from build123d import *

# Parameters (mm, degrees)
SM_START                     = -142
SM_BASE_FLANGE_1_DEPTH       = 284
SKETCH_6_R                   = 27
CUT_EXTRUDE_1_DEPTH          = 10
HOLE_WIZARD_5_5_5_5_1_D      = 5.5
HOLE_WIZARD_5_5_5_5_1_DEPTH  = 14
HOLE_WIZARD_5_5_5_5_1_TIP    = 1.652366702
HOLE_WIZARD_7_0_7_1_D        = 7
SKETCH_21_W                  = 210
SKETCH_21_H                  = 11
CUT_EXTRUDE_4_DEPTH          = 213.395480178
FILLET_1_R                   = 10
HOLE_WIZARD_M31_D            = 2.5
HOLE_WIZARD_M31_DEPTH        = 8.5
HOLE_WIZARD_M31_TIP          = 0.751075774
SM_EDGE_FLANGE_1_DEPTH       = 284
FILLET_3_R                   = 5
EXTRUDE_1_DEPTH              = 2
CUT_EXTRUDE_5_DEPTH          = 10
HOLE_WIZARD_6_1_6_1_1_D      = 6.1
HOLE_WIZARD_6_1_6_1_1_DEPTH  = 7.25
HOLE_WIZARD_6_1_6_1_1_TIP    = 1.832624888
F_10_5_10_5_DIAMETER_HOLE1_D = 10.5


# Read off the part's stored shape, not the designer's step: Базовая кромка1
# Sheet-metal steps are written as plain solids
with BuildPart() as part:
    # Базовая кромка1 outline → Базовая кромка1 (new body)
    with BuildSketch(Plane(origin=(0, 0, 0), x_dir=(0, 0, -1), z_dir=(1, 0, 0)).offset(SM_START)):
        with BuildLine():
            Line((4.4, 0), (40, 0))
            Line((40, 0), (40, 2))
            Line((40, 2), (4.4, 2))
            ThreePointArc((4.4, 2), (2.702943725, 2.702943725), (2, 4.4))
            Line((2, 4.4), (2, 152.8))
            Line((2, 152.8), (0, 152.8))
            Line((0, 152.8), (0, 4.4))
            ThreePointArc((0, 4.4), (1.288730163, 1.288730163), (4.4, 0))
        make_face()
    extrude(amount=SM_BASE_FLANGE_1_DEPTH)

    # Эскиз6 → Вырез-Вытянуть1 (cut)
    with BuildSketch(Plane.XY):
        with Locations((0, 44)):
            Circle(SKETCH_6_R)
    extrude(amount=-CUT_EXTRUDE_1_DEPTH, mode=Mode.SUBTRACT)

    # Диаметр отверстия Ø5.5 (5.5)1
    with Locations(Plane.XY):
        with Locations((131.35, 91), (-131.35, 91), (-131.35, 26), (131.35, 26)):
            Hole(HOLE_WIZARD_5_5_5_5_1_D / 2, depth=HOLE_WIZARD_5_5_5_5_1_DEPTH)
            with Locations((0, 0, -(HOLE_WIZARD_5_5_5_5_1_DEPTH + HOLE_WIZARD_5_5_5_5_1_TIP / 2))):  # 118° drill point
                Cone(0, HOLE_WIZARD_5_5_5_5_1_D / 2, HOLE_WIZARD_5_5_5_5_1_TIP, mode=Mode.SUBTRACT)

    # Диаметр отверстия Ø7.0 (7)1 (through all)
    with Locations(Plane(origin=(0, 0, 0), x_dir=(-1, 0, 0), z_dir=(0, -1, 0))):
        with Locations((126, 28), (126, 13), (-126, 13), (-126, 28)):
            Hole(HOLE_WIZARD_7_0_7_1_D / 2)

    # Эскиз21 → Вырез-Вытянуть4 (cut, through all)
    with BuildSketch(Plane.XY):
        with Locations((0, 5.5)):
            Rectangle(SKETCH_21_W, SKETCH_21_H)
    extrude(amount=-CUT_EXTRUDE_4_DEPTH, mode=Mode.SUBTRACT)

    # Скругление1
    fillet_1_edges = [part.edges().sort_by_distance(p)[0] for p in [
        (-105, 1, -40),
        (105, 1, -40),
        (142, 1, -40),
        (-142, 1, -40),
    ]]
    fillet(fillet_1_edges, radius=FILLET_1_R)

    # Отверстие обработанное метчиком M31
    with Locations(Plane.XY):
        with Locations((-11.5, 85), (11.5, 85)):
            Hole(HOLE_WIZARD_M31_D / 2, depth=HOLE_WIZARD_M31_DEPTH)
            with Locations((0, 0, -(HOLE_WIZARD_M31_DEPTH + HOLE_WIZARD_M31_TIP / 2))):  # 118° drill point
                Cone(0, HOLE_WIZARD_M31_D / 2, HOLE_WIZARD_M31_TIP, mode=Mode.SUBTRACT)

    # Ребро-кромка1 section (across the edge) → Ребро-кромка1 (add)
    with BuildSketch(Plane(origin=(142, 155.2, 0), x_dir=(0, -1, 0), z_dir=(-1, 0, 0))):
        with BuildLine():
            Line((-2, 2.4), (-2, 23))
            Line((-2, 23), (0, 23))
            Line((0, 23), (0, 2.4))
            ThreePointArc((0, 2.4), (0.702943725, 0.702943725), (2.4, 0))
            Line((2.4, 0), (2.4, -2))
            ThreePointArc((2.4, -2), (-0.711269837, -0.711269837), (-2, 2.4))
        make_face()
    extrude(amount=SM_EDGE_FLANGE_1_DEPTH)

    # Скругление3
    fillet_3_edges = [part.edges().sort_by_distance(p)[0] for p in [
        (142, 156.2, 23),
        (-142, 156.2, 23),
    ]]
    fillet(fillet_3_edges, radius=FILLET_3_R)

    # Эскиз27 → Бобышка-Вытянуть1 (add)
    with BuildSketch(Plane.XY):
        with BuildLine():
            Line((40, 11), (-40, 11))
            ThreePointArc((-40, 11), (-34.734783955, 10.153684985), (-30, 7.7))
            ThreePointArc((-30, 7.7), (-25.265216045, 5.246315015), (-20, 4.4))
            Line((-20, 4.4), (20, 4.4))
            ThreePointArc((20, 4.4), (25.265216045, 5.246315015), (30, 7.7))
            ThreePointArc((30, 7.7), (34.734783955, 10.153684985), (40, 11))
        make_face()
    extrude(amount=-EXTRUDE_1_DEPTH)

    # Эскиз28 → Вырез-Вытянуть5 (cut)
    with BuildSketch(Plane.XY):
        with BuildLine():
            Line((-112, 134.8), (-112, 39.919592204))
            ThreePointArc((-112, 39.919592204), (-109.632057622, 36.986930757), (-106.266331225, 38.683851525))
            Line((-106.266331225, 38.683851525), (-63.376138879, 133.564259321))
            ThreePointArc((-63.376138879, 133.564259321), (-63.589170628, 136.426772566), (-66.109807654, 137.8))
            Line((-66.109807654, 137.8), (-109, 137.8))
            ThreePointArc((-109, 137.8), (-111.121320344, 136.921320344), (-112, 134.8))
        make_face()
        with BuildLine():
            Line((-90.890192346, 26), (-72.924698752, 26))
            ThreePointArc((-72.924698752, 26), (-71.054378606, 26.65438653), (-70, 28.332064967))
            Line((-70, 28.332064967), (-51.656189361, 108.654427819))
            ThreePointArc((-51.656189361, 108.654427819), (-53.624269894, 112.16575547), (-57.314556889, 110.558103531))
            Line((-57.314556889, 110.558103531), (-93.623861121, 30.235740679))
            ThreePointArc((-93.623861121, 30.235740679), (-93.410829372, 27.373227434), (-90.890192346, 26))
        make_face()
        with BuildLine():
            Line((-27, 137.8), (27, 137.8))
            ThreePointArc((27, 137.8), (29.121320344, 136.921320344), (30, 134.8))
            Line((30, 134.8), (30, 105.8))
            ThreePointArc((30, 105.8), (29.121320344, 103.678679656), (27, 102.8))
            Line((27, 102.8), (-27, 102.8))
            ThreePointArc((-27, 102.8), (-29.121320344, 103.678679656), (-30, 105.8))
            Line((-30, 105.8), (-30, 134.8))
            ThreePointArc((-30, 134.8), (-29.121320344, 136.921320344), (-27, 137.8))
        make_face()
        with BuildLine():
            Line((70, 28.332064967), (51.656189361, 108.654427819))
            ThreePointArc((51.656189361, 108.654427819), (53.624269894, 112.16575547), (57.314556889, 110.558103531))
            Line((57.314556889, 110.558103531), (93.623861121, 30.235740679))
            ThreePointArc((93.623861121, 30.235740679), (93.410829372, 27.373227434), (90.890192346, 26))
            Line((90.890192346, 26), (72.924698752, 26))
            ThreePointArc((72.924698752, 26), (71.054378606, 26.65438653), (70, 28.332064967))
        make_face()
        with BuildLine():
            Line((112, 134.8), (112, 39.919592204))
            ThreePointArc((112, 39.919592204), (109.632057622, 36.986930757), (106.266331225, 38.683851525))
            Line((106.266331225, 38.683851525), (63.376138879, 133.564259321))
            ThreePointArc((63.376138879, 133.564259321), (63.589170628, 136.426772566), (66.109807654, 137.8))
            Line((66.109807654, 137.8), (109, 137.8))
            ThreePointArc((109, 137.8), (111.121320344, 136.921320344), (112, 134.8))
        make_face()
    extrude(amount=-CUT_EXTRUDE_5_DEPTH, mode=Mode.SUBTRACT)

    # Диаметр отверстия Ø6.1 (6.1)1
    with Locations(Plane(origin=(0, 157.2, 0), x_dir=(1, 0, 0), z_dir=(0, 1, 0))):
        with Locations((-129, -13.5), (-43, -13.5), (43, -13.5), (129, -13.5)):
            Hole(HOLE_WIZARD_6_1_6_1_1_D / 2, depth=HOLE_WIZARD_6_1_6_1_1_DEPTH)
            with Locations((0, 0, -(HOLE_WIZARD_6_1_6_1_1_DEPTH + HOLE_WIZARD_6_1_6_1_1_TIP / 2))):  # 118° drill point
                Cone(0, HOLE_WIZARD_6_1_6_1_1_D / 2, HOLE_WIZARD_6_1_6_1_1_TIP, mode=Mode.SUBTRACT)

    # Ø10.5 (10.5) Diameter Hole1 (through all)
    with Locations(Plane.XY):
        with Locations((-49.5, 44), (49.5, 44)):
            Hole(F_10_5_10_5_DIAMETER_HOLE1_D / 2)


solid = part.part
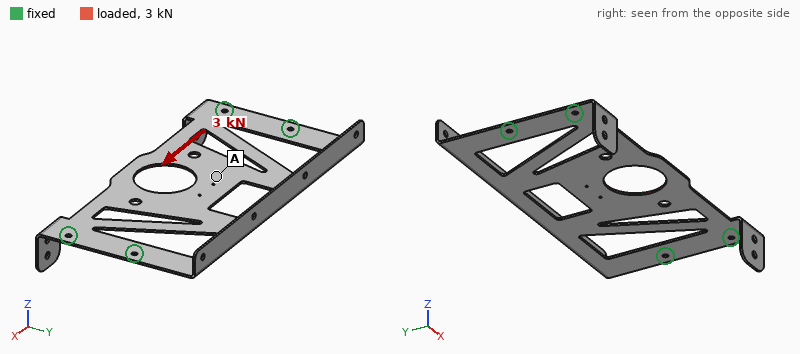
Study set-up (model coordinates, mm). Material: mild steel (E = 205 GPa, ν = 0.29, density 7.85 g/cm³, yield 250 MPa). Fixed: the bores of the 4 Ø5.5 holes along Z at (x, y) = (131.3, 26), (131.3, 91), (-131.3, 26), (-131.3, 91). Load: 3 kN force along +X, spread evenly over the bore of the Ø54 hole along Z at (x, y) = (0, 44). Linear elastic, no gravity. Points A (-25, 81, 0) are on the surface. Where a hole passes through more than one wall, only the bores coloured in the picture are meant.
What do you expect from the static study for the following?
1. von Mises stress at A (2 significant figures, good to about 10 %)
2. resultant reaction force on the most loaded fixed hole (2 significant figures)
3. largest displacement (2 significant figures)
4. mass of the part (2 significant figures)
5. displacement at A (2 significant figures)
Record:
8.9 MPa
1.3 kN
30 µm
600 g
29 µm
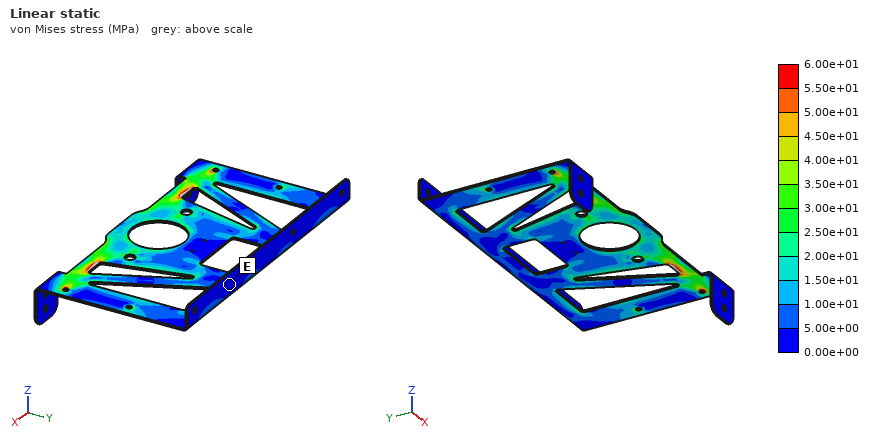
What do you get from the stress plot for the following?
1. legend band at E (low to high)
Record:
0.00e+00 to 5.00e+00 MPa
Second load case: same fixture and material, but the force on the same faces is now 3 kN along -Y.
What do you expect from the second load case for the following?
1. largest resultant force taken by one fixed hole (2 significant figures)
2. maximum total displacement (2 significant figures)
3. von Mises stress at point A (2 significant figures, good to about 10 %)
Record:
980 N
81 µm
17 MPa
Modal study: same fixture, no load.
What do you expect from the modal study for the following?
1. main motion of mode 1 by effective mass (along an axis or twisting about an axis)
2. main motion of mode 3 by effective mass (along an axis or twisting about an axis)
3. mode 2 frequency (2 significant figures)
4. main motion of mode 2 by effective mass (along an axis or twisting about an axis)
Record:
along Z
twisting about Y
160 Hz
along Z
